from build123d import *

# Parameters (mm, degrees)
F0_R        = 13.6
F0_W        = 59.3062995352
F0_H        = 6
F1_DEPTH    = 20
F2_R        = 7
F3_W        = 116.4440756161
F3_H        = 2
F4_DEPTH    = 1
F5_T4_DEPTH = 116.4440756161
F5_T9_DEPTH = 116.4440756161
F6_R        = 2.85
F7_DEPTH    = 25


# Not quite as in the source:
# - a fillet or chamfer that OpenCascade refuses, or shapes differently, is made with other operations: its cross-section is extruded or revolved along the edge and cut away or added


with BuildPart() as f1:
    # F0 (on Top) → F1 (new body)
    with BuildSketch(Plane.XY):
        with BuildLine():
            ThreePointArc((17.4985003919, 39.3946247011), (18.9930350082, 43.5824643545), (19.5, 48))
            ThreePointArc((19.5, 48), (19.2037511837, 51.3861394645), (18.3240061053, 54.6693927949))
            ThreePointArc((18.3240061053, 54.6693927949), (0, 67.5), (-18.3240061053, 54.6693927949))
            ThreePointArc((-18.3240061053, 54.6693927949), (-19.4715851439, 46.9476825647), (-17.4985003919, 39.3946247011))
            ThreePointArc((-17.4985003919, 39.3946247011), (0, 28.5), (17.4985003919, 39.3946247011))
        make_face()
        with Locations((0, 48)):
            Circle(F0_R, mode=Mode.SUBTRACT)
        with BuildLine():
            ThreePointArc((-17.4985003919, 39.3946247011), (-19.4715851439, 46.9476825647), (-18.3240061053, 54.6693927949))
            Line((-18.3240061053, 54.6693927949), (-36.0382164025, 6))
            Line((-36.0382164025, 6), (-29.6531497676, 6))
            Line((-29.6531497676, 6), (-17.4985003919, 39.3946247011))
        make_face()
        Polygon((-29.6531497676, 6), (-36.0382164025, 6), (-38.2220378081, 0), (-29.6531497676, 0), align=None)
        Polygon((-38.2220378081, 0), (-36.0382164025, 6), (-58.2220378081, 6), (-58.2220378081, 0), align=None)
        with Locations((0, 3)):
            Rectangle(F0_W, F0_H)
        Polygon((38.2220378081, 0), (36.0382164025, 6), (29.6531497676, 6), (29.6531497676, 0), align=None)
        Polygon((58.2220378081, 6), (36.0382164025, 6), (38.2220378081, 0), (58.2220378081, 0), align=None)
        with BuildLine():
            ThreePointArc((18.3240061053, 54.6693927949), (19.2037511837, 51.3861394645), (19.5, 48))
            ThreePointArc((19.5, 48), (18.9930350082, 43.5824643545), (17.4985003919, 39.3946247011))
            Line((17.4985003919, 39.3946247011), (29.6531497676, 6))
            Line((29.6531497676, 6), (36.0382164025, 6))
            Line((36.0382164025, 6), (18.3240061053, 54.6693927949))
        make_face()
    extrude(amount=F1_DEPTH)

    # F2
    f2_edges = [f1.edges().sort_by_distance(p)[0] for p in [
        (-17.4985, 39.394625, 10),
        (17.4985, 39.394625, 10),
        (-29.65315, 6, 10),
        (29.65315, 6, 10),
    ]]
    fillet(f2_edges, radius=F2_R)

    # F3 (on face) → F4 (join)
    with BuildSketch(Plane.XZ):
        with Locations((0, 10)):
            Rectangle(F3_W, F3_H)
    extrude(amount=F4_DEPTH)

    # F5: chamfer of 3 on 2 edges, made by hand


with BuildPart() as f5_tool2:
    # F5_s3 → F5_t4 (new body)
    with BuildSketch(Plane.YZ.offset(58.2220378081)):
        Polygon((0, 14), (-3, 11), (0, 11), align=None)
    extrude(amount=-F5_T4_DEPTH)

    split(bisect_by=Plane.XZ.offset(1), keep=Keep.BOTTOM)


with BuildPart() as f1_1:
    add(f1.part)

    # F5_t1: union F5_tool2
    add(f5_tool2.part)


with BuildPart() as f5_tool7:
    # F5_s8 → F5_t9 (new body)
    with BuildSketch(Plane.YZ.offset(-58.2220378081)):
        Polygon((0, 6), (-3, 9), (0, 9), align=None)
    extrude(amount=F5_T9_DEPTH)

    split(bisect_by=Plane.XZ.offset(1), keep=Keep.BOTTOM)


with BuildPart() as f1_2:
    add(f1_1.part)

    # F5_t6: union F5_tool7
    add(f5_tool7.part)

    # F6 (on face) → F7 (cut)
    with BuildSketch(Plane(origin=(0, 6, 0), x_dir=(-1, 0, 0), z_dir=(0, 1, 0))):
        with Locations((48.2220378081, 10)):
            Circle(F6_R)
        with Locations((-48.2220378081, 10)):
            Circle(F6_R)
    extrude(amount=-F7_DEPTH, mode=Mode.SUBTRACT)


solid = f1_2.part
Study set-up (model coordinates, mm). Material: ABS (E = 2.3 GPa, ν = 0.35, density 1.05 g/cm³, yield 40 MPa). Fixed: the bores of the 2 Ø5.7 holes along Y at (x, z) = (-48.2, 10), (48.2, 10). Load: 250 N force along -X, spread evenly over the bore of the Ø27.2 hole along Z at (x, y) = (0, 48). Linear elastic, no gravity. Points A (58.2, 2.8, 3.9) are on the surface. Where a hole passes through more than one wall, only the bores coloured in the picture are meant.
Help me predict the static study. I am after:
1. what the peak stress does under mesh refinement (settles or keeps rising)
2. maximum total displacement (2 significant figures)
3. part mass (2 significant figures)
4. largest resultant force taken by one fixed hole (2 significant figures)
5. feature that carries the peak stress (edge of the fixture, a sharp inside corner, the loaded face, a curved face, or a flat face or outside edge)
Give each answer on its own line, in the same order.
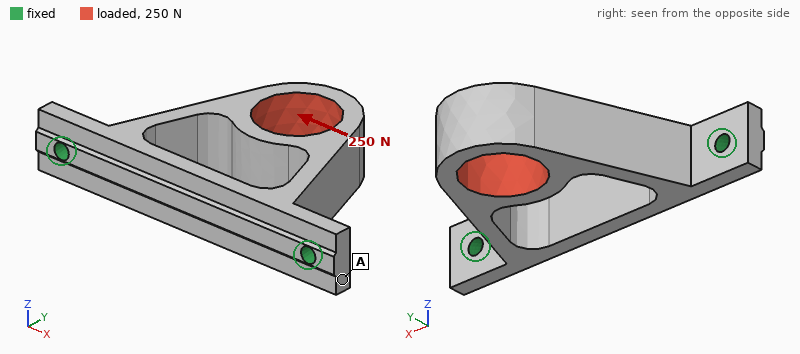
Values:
keeps rising
0.31 mm
40 g
180 N
edge of the fixture
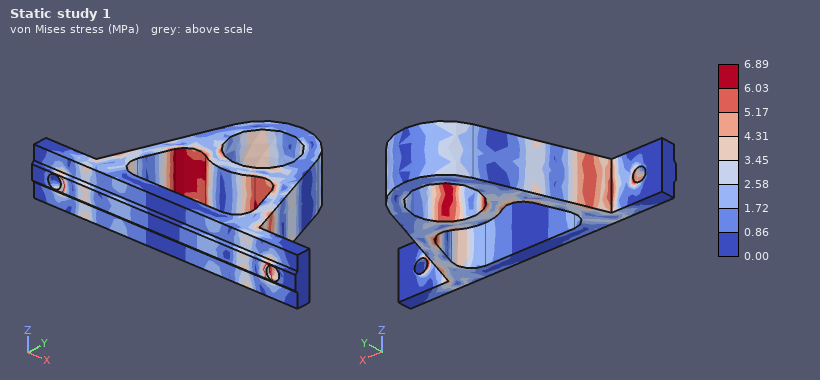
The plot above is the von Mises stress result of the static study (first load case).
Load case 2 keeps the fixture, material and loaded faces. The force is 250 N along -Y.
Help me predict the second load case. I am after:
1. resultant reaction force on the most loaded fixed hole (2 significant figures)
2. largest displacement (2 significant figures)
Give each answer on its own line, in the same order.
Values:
140 N
0.11 mm
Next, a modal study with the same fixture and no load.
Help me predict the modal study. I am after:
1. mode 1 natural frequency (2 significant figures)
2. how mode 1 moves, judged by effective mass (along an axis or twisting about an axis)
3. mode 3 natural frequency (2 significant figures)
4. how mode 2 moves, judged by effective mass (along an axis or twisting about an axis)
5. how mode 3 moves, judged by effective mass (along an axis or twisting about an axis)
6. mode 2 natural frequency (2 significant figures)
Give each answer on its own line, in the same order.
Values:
360 Hz
along Z
1300 Hz
along X
along Y
1100 Hz
